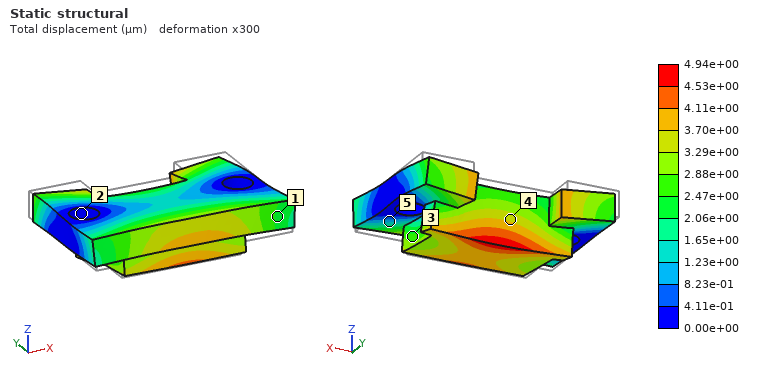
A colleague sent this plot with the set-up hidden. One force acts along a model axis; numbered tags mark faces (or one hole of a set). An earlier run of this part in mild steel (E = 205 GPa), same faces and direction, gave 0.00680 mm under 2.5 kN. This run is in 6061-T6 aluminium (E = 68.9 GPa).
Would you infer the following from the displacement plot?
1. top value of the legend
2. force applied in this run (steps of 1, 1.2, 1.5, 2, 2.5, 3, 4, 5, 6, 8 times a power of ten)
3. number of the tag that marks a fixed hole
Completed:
4.94e+00 µm
600 N
2
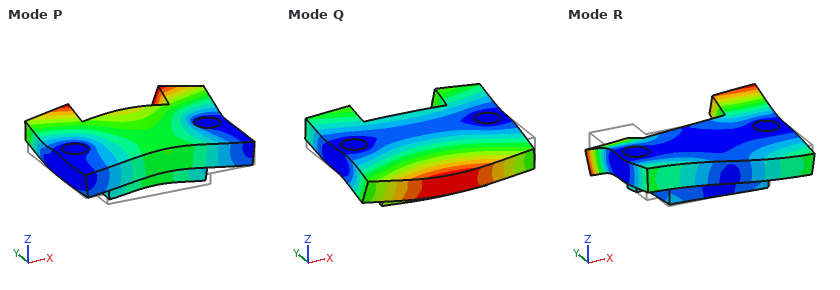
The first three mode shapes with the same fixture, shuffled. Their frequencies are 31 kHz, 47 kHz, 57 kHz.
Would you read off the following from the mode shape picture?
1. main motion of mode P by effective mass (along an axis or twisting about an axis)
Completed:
along Z
